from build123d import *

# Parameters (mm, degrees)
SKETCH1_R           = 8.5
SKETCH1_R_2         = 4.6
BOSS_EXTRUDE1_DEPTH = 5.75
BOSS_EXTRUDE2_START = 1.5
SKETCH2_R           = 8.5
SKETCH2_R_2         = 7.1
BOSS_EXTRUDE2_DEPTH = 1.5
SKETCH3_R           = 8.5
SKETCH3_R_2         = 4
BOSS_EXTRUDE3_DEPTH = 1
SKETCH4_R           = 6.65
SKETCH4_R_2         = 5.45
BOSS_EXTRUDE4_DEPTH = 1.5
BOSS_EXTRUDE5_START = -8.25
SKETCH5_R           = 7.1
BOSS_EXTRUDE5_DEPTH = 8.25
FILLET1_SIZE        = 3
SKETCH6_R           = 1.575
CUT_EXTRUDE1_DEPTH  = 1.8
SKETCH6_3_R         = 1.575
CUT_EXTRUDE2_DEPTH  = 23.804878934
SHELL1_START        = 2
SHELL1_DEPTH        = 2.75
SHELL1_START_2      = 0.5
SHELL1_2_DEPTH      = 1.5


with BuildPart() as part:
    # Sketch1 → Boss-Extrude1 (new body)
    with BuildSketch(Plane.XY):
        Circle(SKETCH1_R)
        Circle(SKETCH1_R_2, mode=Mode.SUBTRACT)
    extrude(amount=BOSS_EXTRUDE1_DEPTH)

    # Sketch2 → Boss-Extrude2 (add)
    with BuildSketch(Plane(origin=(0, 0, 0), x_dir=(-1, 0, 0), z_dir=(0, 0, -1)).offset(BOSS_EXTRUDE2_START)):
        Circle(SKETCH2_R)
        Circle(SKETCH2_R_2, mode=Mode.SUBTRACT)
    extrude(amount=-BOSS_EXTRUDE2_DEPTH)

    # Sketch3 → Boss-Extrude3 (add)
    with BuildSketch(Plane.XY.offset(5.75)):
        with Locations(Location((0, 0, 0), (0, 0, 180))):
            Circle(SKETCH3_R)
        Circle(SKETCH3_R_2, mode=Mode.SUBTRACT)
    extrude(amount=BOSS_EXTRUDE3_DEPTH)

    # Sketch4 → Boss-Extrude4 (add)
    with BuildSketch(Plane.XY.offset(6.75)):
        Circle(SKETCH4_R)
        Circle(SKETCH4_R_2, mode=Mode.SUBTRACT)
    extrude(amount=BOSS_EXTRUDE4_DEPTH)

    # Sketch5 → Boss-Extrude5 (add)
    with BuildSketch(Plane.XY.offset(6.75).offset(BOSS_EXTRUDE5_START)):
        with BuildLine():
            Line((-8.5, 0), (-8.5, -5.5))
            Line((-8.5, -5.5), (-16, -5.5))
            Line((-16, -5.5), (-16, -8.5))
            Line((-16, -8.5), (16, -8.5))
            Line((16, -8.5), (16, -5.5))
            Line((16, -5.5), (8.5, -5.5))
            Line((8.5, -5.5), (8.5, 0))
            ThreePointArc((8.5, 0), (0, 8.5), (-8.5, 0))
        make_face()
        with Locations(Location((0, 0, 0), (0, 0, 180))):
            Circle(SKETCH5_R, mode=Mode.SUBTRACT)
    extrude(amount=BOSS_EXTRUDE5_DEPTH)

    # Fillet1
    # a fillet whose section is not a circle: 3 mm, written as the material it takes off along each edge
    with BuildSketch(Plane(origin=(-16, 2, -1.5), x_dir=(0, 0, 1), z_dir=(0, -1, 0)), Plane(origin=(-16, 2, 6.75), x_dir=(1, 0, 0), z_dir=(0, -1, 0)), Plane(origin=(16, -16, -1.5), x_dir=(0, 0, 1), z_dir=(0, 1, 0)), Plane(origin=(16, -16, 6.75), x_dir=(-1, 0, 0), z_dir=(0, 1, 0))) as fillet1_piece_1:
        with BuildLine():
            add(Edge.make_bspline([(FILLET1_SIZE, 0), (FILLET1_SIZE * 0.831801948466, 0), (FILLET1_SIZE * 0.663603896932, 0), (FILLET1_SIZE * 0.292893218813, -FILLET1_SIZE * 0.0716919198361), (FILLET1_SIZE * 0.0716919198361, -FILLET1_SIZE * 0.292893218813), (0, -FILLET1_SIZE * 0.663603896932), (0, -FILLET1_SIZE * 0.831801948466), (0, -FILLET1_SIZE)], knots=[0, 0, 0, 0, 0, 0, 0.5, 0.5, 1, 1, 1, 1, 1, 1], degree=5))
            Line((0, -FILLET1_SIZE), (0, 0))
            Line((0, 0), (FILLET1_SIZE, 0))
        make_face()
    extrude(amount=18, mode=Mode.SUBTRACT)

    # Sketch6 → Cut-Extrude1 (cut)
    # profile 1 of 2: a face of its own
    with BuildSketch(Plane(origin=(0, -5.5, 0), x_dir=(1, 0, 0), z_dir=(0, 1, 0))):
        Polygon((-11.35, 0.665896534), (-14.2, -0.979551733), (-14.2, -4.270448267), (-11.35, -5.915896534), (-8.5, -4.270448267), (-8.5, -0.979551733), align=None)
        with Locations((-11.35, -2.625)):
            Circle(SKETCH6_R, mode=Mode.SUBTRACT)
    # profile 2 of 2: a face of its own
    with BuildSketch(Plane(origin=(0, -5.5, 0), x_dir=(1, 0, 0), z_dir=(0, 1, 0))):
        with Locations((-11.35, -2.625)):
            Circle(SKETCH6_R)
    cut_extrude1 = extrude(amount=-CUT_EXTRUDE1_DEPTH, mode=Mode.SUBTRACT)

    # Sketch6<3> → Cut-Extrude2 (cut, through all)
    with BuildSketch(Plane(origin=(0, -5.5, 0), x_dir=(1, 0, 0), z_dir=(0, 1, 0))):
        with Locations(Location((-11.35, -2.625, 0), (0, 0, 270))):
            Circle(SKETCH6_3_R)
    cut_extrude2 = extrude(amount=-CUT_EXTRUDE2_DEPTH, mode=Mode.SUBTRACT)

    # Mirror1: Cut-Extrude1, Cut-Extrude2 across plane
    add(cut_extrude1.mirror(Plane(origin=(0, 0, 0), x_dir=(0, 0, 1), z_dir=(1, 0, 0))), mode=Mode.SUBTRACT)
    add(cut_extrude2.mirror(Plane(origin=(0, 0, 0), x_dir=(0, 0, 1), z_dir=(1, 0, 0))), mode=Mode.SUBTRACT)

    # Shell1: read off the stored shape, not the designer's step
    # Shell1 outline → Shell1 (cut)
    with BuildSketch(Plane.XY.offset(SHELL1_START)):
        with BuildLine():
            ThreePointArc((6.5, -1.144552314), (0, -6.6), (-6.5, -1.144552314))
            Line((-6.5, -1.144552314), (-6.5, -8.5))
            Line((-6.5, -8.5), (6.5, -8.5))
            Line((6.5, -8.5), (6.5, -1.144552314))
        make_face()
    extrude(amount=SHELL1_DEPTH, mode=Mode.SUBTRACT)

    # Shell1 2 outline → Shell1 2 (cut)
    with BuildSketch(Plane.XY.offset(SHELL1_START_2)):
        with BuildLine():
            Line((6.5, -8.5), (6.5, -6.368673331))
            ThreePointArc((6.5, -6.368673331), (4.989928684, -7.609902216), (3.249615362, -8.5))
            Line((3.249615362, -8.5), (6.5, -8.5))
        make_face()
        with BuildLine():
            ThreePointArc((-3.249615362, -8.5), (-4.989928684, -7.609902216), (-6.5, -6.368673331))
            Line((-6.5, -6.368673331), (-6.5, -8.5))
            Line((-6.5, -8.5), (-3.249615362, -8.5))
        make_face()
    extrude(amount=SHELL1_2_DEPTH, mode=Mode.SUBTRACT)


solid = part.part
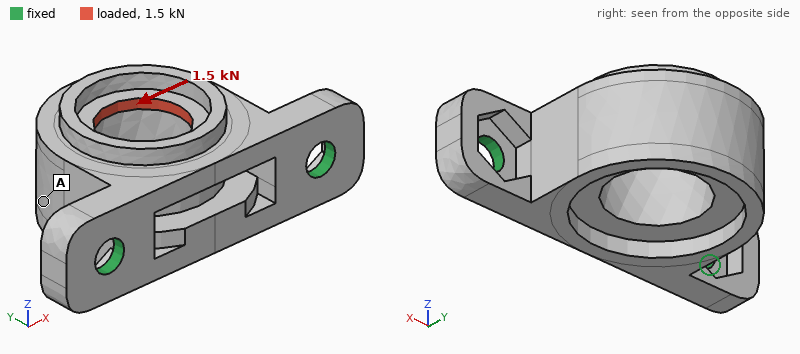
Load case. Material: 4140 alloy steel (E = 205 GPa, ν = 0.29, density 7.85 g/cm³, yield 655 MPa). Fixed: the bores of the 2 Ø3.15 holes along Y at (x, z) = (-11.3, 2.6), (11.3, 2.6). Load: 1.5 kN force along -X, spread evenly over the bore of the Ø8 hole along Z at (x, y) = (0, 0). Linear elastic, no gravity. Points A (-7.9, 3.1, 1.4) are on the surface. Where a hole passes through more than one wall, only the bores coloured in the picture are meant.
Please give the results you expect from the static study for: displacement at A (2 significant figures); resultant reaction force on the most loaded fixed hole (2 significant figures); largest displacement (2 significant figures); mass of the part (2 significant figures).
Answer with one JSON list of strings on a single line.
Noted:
["9.9 µm", "980 N", "14 µm", "13 g"]
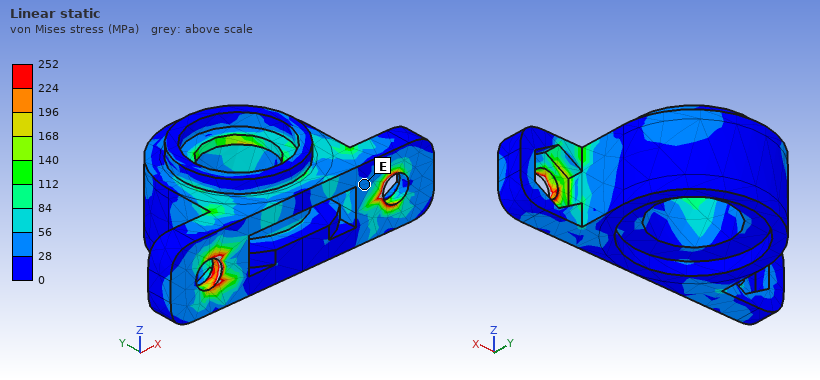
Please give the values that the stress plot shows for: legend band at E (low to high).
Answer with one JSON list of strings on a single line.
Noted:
["28 to 56 MPa"]
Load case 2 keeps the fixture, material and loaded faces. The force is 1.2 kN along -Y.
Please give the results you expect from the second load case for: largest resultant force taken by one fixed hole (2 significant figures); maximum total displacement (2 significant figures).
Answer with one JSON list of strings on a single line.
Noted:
["730 N", "60 µm"]
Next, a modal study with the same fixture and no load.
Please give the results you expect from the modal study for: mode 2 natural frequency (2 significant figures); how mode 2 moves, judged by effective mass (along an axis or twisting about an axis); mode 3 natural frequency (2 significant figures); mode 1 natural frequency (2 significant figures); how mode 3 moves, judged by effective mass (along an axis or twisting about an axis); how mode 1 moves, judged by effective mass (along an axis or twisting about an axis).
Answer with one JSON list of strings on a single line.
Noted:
["19 kHz", "along X", "22 kHz", "5800 Hz", "along Y", "along Z"]
